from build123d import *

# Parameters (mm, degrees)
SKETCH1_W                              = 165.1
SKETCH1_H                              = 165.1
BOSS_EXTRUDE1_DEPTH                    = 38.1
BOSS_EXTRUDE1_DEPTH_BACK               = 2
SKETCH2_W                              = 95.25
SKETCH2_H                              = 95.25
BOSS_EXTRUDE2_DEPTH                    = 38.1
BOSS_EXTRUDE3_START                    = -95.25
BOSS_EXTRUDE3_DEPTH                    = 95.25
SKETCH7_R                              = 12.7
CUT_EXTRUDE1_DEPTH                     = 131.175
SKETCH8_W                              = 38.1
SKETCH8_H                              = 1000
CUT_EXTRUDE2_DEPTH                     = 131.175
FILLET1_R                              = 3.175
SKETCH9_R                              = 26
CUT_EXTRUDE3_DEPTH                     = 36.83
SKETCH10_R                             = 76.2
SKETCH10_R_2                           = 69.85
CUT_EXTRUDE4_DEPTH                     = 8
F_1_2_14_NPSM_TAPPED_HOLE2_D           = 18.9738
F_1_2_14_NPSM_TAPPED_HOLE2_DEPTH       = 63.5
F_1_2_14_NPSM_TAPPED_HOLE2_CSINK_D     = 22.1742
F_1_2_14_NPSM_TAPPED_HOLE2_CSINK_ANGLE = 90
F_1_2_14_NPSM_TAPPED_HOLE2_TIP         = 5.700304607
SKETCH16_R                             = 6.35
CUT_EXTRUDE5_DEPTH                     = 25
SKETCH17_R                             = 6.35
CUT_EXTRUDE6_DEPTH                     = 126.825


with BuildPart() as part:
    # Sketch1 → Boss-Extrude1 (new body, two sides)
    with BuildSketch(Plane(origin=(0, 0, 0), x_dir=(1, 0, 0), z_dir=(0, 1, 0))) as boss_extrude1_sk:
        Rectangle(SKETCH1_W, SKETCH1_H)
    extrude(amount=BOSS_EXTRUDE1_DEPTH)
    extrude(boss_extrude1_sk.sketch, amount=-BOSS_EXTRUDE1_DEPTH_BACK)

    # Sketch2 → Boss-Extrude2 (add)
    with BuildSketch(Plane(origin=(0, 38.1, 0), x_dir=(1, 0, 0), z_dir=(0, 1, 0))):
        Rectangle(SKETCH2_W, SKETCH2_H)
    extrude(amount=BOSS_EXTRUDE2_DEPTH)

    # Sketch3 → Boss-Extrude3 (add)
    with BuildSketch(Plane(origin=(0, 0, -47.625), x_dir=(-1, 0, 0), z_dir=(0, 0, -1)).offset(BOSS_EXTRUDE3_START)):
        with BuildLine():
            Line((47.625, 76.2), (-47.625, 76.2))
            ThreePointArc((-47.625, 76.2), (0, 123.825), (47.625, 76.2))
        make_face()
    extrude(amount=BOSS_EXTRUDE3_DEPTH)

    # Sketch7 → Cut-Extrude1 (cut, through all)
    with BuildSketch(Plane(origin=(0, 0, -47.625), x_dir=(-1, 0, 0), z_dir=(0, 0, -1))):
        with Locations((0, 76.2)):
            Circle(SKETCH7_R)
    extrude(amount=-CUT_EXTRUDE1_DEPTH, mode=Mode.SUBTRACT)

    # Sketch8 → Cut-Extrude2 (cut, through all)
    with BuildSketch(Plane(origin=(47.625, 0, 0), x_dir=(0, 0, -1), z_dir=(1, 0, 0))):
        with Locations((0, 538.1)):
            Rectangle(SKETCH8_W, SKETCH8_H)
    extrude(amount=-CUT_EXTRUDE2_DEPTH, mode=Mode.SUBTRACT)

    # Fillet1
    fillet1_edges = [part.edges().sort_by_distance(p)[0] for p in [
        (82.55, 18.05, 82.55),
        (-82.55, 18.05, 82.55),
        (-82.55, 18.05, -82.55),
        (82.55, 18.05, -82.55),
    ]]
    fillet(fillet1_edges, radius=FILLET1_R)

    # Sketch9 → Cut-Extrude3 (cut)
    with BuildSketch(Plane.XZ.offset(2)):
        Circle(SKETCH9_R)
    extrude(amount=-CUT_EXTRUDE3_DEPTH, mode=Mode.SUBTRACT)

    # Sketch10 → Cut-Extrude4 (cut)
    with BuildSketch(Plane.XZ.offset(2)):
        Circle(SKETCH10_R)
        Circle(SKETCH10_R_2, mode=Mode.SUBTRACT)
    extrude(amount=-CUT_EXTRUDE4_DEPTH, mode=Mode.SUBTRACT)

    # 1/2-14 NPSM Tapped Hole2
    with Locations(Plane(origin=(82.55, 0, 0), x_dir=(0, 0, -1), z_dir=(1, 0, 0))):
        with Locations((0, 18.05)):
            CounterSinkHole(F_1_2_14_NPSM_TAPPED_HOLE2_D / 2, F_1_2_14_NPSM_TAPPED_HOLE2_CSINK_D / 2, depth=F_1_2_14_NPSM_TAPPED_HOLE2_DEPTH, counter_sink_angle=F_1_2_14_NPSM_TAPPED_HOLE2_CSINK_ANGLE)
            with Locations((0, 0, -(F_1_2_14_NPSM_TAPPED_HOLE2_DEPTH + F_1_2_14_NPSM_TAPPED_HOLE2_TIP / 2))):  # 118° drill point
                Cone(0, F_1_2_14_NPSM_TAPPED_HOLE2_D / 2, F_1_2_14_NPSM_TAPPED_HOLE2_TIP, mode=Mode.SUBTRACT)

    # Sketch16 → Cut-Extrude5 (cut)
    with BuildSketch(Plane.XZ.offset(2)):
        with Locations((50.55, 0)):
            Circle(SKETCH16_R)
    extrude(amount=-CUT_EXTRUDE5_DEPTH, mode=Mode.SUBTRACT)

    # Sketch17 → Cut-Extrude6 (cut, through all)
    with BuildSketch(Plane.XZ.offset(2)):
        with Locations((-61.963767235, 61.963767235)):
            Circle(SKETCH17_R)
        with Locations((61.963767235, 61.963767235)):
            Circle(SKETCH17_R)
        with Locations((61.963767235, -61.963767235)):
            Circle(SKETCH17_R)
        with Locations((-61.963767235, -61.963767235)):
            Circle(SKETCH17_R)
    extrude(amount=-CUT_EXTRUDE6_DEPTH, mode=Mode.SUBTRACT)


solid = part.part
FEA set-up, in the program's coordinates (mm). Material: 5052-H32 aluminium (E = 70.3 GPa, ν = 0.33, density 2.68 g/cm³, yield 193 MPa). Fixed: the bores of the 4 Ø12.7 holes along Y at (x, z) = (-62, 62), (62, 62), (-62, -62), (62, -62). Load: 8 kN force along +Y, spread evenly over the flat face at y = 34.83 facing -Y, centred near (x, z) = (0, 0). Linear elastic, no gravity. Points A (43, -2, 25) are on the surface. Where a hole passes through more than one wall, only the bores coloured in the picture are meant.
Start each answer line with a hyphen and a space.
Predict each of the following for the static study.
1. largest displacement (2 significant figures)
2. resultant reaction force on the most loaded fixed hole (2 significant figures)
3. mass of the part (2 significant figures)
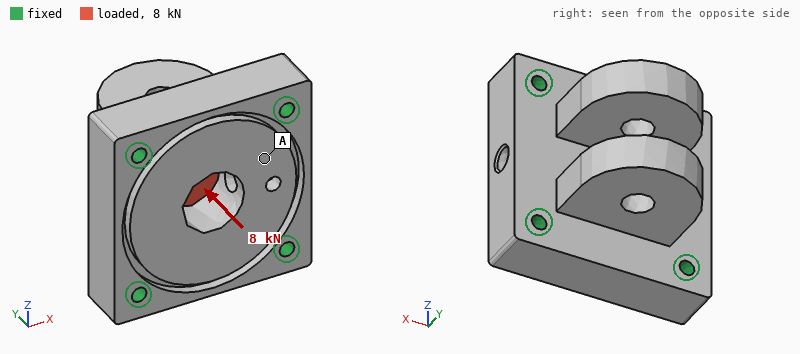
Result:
- 53 µm
- 2.0 kN
- 3.6 kg
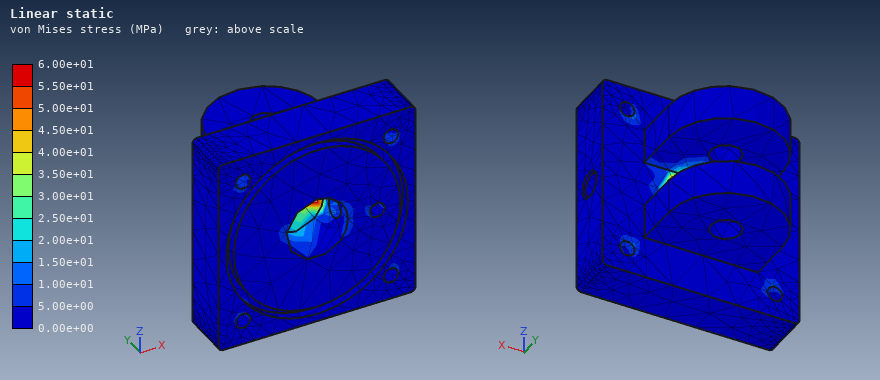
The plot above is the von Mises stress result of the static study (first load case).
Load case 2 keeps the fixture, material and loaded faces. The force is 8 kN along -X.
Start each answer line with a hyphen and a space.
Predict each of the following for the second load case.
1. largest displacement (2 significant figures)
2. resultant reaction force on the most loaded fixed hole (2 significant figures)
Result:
- 7.5 µm
- 2.3 kN
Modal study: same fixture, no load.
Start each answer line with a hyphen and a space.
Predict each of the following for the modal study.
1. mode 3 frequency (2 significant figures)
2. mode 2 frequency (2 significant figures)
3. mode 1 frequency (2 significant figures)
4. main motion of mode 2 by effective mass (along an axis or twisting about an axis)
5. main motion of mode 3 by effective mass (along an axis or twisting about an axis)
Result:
- 4800 Hz
- 2700 Hz
- 2600 Hz
- along Z
- along X
